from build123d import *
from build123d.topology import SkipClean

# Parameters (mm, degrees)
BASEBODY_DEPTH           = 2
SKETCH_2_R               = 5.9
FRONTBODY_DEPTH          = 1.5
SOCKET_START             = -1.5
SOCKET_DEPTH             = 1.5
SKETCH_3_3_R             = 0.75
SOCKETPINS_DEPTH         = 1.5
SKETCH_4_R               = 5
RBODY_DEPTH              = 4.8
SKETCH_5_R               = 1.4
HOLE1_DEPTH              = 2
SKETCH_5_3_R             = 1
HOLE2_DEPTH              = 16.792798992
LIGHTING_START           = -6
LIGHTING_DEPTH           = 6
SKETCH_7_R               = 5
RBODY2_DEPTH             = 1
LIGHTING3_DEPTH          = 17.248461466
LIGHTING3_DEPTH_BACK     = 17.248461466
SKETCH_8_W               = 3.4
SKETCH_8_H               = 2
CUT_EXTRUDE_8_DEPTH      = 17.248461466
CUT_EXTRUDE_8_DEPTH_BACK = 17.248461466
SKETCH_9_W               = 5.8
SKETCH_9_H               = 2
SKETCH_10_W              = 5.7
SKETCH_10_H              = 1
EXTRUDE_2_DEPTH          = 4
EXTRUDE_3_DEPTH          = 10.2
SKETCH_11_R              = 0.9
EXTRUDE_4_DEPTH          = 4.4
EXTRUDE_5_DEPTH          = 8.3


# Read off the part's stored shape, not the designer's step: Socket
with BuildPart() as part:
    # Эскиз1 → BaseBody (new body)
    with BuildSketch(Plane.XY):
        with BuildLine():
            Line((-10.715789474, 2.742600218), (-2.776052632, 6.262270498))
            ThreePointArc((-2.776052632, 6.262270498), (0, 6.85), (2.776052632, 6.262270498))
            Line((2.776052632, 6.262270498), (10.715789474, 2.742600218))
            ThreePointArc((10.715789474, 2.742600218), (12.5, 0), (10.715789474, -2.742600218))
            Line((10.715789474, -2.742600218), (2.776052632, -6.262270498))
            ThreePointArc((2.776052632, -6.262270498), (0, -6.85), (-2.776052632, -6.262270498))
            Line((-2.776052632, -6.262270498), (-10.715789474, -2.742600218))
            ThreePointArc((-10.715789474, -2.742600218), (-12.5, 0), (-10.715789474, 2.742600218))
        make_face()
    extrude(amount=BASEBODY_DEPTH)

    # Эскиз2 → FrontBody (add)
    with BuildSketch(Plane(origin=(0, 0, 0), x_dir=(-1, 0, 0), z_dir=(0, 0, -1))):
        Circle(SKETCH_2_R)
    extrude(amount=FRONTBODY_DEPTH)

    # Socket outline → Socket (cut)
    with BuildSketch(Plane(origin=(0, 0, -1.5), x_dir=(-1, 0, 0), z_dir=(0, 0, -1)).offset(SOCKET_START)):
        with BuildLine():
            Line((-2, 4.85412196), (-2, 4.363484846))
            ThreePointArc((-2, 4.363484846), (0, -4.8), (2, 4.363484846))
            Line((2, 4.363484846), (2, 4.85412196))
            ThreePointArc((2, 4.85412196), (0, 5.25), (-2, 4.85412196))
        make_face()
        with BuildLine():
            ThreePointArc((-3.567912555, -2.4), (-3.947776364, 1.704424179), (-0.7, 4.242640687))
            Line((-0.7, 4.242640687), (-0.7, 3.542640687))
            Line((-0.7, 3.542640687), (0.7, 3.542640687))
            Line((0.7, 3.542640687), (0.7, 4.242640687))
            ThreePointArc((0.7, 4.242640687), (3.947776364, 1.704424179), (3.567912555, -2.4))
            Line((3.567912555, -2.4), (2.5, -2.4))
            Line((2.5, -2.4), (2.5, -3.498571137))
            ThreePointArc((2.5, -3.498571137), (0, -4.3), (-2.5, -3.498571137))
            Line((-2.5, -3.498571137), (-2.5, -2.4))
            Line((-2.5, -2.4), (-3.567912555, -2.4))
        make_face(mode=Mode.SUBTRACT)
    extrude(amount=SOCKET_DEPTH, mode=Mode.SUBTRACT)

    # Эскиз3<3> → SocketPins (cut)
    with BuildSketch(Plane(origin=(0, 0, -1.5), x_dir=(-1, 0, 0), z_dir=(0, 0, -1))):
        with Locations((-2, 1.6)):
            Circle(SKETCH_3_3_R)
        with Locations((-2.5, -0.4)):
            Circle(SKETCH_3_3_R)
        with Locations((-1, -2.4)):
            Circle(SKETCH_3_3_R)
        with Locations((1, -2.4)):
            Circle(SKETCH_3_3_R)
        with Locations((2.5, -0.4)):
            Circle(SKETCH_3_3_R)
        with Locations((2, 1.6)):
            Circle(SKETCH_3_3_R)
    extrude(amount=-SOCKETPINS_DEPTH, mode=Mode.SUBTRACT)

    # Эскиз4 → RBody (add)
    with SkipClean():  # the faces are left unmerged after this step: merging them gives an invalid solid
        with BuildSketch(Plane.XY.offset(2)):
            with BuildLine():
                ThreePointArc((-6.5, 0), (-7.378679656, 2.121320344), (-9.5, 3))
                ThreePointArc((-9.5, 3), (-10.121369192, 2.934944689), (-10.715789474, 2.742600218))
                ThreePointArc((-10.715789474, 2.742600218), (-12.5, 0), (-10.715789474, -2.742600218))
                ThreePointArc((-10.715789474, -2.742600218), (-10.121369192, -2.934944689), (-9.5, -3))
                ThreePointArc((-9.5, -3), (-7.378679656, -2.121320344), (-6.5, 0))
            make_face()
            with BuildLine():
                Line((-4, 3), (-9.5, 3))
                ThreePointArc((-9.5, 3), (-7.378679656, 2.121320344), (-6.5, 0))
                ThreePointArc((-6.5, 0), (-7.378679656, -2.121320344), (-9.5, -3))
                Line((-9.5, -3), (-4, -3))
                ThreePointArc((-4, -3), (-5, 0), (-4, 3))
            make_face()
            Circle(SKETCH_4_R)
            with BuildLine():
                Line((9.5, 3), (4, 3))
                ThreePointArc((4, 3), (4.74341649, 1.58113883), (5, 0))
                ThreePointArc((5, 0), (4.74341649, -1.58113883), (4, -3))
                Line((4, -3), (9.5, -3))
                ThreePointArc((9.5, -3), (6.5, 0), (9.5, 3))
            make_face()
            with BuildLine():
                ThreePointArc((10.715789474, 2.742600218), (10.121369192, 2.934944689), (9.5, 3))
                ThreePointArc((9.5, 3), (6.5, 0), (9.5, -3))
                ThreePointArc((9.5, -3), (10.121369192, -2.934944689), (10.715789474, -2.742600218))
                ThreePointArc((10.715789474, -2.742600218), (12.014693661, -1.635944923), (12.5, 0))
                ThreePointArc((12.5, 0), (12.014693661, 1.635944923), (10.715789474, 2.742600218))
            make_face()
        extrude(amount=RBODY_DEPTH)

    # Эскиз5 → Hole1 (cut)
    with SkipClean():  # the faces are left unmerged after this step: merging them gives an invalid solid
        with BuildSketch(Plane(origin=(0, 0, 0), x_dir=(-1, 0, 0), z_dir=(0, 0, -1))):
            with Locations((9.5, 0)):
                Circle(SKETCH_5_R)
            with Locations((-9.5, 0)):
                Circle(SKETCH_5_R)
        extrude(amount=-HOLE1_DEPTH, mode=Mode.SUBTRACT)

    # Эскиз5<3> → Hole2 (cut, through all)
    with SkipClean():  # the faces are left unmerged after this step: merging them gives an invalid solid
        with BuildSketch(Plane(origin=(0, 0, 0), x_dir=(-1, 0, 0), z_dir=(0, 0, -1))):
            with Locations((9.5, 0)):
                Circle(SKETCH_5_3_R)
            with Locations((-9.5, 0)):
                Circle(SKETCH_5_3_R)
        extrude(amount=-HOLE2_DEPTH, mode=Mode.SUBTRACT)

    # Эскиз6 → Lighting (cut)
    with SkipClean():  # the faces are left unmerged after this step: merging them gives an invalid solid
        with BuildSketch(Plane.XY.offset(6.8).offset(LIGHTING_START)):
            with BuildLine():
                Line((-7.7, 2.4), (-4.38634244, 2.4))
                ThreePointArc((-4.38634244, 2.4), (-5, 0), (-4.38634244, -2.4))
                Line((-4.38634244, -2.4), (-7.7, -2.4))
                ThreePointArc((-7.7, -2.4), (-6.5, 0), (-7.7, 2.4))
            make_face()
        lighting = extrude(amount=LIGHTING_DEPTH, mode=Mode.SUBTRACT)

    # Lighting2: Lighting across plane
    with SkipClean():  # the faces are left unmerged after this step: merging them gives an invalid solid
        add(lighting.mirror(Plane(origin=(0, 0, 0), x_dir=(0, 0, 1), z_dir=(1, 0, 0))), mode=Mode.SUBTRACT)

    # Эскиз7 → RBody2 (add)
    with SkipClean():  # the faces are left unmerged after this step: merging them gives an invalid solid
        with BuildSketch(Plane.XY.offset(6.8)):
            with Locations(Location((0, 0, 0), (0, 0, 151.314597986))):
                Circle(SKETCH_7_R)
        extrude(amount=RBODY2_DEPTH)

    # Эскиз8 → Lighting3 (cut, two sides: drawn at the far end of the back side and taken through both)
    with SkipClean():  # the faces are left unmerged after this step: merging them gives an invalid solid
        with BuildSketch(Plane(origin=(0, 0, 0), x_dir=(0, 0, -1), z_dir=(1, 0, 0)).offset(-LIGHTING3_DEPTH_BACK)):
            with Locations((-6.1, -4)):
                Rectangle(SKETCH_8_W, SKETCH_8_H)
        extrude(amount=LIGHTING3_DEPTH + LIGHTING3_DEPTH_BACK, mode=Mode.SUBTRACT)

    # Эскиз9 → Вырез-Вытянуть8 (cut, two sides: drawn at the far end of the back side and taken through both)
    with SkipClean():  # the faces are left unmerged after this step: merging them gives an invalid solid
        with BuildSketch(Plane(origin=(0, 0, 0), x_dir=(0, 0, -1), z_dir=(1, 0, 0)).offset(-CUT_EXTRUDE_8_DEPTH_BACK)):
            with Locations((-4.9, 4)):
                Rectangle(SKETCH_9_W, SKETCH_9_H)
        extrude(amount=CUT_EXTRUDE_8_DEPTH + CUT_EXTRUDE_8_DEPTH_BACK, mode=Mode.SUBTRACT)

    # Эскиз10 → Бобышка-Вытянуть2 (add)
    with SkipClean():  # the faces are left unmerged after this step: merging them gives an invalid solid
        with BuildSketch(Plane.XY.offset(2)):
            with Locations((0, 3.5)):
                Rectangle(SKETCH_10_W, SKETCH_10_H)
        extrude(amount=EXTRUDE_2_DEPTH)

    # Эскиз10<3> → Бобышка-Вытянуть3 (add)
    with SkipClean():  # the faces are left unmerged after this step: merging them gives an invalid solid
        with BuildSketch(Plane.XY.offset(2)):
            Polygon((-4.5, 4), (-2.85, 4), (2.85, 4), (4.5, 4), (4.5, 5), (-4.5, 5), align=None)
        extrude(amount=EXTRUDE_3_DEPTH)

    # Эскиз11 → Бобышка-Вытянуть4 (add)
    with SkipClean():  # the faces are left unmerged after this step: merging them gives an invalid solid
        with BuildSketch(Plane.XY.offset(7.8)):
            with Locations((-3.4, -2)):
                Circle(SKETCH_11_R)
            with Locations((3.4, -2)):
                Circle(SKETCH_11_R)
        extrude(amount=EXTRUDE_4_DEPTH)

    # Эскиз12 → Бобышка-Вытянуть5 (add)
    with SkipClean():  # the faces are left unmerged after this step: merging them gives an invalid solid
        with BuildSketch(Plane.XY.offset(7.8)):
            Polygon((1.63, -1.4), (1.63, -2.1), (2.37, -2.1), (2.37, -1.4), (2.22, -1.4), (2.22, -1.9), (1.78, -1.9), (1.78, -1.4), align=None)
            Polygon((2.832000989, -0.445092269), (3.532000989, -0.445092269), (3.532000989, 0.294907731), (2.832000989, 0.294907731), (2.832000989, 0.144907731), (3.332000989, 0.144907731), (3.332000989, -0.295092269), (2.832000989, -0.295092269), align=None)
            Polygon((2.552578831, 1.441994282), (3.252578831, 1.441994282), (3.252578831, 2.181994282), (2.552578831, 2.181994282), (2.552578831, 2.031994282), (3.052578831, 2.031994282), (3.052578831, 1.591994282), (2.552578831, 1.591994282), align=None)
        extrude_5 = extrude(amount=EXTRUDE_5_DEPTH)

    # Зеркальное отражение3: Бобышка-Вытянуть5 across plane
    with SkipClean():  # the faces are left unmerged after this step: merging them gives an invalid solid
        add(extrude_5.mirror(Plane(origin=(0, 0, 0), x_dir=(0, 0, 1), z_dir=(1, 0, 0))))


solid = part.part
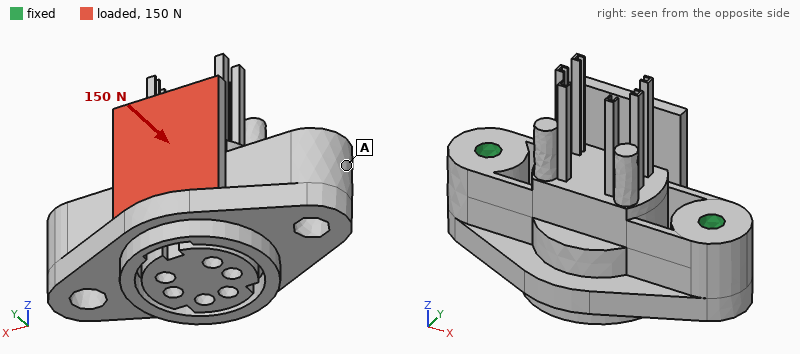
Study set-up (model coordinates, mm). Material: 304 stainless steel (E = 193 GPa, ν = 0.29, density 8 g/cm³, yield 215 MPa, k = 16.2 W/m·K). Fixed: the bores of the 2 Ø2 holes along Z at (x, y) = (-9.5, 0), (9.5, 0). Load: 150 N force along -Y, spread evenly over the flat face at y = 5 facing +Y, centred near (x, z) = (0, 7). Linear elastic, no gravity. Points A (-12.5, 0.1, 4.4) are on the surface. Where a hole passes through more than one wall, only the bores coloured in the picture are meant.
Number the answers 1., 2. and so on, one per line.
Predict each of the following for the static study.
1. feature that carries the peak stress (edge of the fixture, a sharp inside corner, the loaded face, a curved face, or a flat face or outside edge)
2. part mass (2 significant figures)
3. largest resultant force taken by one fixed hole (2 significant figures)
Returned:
1. the loaded face
2. 11 g
3. 75 N
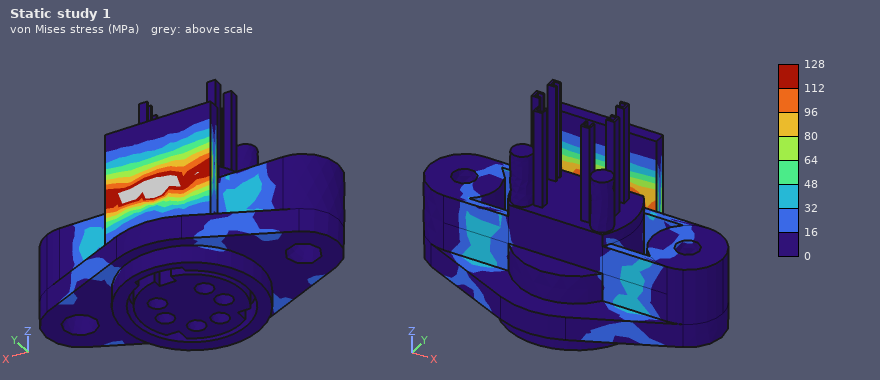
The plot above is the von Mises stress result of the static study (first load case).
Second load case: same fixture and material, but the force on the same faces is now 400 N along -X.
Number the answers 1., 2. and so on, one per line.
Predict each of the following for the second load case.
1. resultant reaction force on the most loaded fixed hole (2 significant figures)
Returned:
1. 240 N
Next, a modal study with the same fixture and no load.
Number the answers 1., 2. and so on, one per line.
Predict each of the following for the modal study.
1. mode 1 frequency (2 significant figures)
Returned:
1. 8000 Hz
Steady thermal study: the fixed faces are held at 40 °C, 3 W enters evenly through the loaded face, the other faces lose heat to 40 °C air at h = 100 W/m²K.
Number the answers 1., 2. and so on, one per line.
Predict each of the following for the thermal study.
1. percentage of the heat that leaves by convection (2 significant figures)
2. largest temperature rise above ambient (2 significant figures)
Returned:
1. 58 %
2. 66 K
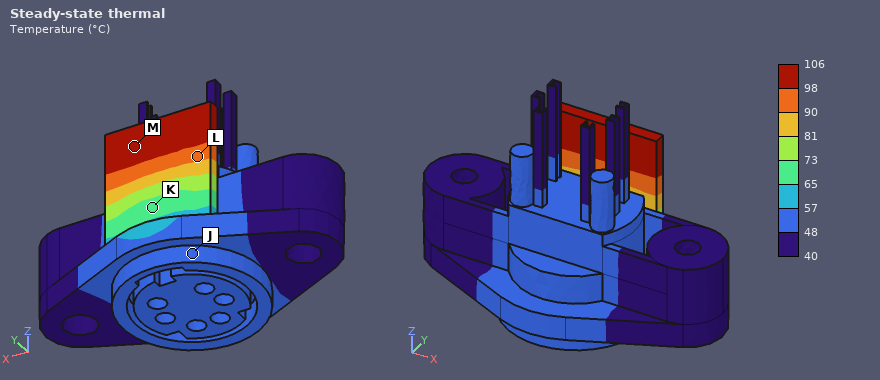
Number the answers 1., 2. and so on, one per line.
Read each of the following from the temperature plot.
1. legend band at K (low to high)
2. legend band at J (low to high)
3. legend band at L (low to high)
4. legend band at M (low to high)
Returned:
1. 65 to 73 °C
2. 48 to 57 °C
3. 90 to 98 °C
4. 98 to 106 °C
